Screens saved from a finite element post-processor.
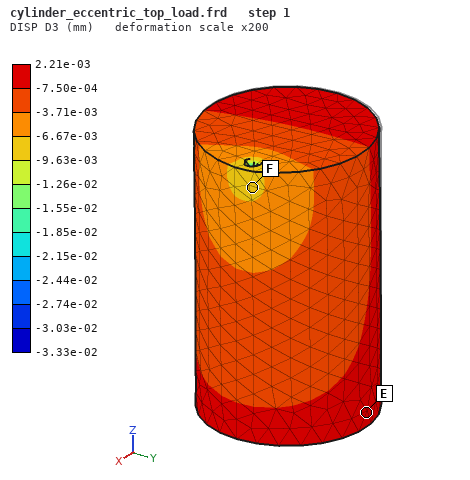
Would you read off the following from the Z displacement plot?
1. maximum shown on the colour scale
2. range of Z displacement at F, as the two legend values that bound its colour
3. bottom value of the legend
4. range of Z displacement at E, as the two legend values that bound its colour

2.21e-03 mm
-9.63e-03 to -6.67e-03 mm
-3.33e-02 mm
-7.50e-04 to 2.21e-03 mm
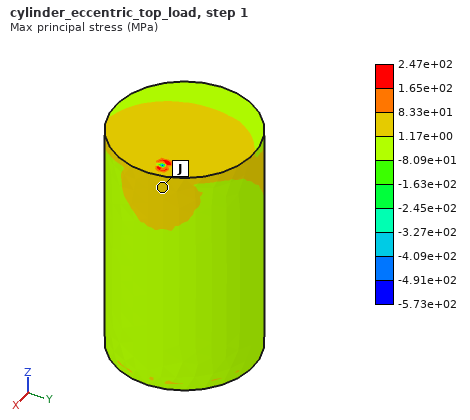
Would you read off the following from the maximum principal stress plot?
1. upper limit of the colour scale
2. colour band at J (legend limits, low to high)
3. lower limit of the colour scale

2.47e+02 MPa
1.17e+00 to 8.33e+01 MPa
-5.73e+02 MPa
